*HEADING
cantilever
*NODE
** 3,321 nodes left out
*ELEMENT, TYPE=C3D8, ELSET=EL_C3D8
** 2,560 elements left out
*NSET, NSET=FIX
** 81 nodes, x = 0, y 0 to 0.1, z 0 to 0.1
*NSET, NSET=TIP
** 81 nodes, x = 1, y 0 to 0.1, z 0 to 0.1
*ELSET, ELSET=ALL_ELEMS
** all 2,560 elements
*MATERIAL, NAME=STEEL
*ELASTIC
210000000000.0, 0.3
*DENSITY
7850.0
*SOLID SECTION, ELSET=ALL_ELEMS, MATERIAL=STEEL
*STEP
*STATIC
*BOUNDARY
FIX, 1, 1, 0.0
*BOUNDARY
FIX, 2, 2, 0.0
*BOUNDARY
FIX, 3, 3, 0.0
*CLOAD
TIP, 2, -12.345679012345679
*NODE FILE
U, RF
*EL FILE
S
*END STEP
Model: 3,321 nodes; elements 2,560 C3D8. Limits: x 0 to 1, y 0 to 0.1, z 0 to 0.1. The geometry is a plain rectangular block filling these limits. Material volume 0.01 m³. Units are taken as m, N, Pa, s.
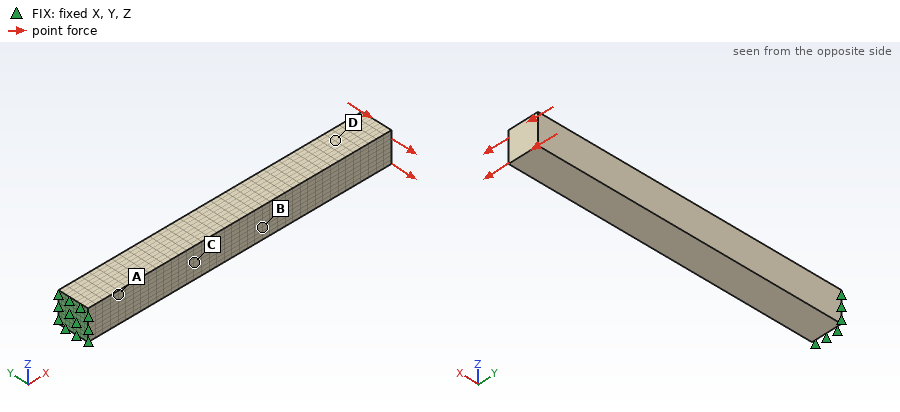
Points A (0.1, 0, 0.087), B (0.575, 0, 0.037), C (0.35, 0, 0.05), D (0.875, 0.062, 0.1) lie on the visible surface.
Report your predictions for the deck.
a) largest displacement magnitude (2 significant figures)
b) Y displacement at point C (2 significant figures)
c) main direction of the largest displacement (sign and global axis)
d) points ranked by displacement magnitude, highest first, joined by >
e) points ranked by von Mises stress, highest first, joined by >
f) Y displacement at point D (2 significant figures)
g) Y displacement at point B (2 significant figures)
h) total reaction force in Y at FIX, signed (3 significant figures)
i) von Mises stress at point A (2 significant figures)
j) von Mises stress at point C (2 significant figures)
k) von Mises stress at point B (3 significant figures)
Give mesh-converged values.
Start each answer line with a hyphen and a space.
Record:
- 1.9e-04 m
- -3.1e-05 m
- -Y
- D > B > C > A
- A > C > B > D
- -1.5e-04 m
- -7.6e-05 m
- 1000 N
- 5.4e+06 Pa
- 3.9e+06 Pa
- 2.55e+06 Pa
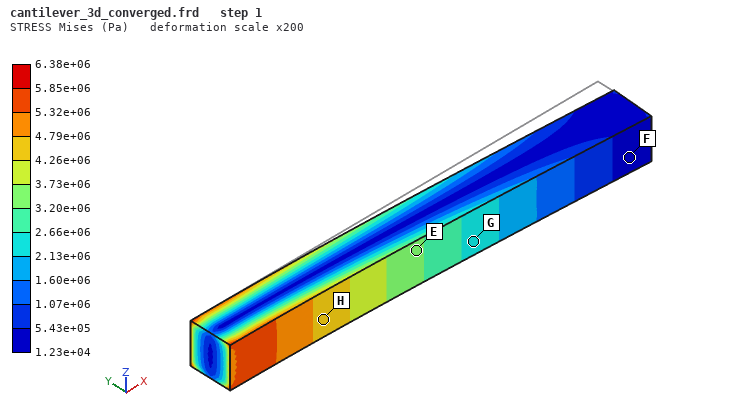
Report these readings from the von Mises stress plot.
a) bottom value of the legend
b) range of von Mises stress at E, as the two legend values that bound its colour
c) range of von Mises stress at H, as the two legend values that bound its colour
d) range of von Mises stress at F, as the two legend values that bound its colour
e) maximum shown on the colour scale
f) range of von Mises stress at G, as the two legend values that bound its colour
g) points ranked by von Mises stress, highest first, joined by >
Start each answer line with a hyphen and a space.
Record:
- 1.23e+04 Pa
- 3.20e+06 to 3.73e+06 Pa
- 4.26e+06 to 4.79e+06 Pa
- 1.23e+04 to 5.43e+05 Pa
- 6.38e+06 Pa
- 2.13e+06 to 2.66e+06 Pa
- H > E > G > F
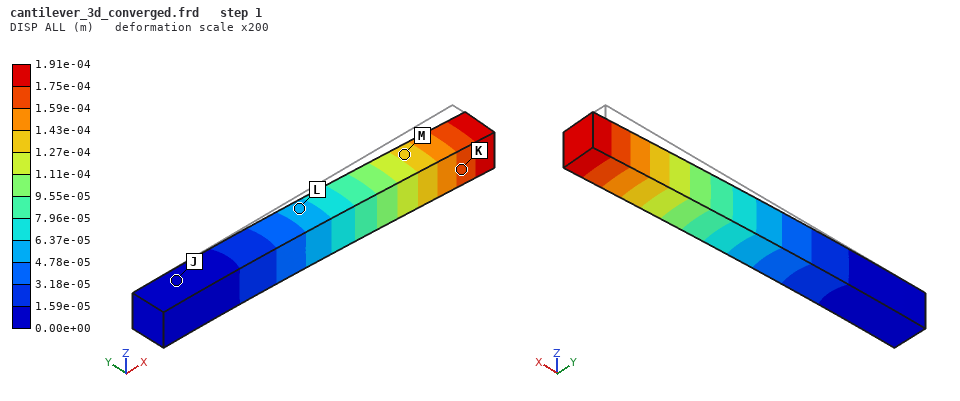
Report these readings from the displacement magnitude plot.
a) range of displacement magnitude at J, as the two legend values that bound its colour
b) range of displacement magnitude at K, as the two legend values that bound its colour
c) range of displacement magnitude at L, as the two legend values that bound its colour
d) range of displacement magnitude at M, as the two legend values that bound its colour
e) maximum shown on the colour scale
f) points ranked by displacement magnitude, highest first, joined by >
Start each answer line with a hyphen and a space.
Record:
- 0.00e+00 to 1.59e-05 m
- 1.59e-04 to 1.75e-04 m
- 4.78e-05 to 6.37e-05 m
- 1.27e-04 to 1.43e-04 m
- 1.91e-04 m
- K > M > L > J
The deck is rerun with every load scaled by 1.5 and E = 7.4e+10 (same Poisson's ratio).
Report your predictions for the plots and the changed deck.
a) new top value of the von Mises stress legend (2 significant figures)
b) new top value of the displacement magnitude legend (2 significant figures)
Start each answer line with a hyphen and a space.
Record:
- 9.6e+06 Pa
- 8.1e-04 m
